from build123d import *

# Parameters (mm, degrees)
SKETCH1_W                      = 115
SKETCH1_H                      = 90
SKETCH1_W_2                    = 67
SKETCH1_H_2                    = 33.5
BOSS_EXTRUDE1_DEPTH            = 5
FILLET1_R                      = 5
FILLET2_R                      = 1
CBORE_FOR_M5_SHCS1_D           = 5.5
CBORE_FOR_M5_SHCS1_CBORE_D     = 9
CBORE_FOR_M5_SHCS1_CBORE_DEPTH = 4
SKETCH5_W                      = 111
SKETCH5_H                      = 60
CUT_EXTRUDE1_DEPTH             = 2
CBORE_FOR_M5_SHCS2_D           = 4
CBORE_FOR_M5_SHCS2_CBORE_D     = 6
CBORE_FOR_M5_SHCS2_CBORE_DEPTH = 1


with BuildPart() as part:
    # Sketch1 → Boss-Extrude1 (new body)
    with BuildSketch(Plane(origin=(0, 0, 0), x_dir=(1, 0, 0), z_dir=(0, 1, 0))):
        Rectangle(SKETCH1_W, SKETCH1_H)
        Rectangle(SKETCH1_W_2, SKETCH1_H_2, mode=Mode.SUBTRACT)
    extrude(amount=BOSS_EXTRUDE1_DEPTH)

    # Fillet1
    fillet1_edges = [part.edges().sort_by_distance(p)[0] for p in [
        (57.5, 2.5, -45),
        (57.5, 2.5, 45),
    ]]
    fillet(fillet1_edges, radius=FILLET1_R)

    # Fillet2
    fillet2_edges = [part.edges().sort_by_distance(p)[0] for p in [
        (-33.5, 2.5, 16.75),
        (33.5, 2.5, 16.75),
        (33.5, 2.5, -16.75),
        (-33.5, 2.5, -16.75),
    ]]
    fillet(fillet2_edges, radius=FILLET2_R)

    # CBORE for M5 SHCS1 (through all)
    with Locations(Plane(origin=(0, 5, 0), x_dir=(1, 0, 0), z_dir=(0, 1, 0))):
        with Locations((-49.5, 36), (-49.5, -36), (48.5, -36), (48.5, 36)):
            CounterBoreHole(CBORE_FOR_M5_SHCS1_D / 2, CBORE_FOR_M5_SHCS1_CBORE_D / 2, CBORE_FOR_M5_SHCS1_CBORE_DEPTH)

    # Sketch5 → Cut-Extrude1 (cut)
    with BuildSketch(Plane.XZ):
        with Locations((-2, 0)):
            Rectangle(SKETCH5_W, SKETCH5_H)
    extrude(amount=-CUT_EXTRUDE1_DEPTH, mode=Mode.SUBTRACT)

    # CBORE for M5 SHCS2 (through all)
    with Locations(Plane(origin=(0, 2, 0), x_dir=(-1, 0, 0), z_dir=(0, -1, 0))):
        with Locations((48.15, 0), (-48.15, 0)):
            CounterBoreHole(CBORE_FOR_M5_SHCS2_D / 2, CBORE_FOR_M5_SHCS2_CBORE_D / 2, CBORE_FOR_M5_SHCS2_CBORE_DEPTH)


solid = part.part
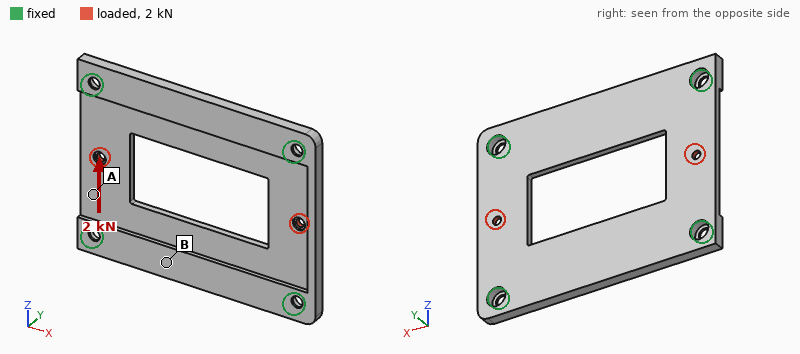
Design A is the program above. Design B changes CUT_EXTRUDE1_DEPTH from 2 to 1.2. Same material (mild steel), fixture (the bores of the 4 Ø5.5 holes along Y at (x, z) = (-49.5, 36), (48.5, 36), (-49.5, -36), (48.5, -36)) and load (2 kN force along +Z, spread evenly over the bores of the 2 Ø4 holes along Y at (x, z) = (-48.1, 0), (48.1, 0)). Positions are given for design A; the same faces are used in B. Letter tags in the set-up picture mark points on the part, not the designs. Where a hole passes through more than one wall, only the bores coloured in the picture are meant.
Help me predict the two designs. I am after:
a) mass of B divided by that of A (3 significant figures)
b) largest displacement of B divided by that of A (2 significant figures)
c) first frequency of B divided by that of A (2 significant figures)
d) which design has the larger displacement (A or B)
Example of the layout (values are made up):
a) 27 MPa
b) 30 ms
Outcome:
a) 1.11
b) 0.52
c) 0.99
d) A
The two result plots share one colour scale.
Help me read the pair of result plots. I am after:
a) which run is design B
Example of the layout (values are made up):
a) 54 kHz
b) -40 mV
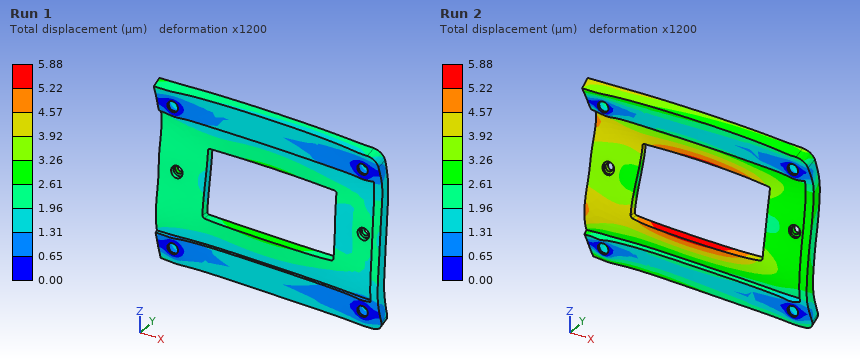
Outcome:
a) Run 1
